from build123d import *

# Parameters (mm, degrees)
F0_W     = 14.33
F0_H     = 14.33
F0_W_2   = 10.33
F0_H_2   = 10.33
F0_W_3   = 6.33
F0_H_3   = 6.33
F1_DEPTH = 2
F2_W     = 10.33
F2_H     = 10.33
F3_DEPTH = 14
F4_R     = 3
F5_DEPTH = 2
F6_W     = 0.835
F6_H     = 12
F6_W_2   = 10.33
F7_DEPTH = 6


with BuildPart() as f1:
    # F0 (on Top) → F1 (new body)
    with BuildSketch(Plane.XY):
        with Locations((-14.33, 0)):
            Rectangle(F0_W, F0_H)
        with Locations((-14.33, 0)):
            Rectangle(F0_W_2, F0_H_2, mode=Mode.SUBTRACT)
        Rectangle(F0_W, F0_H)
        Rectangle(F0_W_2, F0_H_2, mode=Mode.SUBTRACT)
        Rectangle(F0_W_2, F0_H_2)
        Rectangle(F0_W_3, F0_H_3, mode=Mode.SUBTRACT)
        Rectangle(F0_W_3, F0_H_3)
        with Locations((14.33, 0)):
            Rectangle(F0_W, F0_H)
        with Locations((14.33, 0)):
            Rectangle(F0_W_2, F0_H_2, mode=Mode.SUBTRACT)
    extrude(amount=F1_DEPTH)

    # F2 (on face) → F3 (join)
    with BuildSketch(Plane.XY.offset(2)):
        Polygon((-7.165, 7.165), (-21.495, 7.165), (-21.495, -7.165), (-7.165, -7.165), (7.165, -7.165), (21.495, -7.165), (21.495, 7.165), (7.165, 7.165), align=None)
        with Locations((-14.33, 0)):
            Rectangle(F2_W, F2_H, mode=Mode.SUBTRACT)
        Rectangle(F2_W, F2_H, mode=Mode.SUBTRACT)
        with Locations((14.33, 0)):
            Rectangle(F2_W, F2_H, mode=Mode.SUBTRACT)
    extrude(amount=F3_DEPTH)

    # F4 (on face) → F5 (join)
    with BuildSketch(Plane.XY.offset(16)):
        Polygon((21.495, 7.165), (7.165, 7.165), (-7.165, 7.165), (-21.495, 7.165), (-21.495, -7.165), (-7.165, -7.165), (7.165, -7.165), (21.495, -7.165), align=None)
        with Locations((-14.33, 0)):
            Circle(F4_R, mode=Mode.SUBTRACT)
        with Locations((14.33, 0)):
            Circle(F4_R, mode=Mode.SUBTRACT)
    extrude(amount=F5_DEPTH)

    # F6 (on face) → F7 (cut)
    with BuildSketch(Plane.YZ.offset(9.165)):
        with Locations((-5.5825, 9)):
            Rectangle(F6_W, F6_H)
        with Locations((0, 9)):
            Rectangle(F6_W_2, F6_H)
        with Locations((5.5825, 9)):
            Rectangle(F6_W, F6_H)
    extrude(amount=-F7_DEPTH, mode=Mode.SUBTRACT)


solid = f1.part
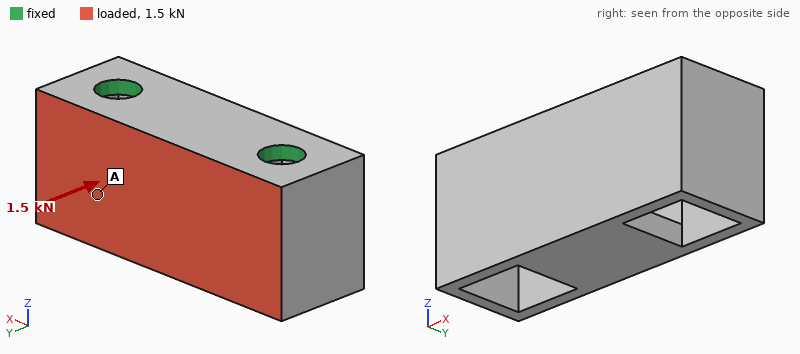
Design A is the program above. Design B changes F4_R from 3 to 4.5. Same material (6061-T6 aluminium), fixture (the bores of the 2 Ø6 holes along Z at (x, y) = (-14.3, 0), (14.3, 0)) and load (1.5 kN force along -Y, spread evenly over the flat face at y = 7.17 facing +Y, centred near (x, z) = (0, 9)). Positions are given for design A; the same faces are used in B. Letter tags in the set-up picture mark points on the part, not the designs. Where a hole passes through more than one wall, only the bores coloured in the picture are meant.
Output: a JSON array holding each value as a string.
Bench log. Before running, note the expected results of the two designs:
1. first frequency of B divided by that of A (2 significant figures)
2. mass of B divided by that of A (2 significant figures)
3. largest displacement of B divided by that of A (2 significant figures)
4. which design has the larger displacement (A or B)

["1.5", "0.97", "0.48", "A"]
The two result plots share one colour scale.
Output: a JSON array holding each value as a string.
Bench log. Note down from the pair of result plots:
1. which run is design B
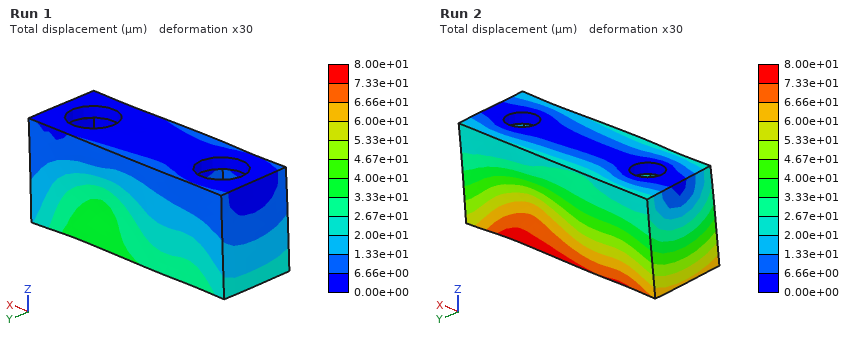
["Run 1"]
